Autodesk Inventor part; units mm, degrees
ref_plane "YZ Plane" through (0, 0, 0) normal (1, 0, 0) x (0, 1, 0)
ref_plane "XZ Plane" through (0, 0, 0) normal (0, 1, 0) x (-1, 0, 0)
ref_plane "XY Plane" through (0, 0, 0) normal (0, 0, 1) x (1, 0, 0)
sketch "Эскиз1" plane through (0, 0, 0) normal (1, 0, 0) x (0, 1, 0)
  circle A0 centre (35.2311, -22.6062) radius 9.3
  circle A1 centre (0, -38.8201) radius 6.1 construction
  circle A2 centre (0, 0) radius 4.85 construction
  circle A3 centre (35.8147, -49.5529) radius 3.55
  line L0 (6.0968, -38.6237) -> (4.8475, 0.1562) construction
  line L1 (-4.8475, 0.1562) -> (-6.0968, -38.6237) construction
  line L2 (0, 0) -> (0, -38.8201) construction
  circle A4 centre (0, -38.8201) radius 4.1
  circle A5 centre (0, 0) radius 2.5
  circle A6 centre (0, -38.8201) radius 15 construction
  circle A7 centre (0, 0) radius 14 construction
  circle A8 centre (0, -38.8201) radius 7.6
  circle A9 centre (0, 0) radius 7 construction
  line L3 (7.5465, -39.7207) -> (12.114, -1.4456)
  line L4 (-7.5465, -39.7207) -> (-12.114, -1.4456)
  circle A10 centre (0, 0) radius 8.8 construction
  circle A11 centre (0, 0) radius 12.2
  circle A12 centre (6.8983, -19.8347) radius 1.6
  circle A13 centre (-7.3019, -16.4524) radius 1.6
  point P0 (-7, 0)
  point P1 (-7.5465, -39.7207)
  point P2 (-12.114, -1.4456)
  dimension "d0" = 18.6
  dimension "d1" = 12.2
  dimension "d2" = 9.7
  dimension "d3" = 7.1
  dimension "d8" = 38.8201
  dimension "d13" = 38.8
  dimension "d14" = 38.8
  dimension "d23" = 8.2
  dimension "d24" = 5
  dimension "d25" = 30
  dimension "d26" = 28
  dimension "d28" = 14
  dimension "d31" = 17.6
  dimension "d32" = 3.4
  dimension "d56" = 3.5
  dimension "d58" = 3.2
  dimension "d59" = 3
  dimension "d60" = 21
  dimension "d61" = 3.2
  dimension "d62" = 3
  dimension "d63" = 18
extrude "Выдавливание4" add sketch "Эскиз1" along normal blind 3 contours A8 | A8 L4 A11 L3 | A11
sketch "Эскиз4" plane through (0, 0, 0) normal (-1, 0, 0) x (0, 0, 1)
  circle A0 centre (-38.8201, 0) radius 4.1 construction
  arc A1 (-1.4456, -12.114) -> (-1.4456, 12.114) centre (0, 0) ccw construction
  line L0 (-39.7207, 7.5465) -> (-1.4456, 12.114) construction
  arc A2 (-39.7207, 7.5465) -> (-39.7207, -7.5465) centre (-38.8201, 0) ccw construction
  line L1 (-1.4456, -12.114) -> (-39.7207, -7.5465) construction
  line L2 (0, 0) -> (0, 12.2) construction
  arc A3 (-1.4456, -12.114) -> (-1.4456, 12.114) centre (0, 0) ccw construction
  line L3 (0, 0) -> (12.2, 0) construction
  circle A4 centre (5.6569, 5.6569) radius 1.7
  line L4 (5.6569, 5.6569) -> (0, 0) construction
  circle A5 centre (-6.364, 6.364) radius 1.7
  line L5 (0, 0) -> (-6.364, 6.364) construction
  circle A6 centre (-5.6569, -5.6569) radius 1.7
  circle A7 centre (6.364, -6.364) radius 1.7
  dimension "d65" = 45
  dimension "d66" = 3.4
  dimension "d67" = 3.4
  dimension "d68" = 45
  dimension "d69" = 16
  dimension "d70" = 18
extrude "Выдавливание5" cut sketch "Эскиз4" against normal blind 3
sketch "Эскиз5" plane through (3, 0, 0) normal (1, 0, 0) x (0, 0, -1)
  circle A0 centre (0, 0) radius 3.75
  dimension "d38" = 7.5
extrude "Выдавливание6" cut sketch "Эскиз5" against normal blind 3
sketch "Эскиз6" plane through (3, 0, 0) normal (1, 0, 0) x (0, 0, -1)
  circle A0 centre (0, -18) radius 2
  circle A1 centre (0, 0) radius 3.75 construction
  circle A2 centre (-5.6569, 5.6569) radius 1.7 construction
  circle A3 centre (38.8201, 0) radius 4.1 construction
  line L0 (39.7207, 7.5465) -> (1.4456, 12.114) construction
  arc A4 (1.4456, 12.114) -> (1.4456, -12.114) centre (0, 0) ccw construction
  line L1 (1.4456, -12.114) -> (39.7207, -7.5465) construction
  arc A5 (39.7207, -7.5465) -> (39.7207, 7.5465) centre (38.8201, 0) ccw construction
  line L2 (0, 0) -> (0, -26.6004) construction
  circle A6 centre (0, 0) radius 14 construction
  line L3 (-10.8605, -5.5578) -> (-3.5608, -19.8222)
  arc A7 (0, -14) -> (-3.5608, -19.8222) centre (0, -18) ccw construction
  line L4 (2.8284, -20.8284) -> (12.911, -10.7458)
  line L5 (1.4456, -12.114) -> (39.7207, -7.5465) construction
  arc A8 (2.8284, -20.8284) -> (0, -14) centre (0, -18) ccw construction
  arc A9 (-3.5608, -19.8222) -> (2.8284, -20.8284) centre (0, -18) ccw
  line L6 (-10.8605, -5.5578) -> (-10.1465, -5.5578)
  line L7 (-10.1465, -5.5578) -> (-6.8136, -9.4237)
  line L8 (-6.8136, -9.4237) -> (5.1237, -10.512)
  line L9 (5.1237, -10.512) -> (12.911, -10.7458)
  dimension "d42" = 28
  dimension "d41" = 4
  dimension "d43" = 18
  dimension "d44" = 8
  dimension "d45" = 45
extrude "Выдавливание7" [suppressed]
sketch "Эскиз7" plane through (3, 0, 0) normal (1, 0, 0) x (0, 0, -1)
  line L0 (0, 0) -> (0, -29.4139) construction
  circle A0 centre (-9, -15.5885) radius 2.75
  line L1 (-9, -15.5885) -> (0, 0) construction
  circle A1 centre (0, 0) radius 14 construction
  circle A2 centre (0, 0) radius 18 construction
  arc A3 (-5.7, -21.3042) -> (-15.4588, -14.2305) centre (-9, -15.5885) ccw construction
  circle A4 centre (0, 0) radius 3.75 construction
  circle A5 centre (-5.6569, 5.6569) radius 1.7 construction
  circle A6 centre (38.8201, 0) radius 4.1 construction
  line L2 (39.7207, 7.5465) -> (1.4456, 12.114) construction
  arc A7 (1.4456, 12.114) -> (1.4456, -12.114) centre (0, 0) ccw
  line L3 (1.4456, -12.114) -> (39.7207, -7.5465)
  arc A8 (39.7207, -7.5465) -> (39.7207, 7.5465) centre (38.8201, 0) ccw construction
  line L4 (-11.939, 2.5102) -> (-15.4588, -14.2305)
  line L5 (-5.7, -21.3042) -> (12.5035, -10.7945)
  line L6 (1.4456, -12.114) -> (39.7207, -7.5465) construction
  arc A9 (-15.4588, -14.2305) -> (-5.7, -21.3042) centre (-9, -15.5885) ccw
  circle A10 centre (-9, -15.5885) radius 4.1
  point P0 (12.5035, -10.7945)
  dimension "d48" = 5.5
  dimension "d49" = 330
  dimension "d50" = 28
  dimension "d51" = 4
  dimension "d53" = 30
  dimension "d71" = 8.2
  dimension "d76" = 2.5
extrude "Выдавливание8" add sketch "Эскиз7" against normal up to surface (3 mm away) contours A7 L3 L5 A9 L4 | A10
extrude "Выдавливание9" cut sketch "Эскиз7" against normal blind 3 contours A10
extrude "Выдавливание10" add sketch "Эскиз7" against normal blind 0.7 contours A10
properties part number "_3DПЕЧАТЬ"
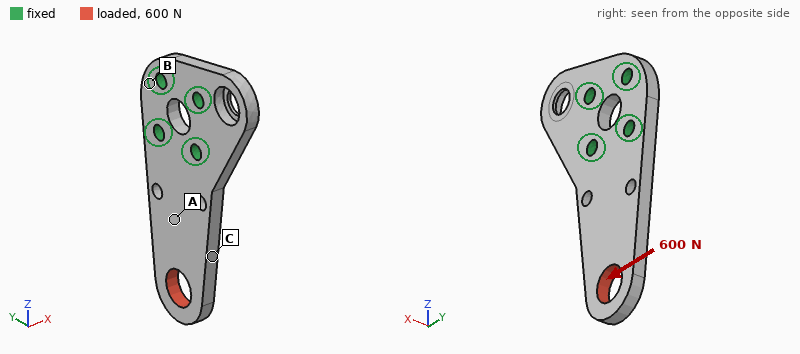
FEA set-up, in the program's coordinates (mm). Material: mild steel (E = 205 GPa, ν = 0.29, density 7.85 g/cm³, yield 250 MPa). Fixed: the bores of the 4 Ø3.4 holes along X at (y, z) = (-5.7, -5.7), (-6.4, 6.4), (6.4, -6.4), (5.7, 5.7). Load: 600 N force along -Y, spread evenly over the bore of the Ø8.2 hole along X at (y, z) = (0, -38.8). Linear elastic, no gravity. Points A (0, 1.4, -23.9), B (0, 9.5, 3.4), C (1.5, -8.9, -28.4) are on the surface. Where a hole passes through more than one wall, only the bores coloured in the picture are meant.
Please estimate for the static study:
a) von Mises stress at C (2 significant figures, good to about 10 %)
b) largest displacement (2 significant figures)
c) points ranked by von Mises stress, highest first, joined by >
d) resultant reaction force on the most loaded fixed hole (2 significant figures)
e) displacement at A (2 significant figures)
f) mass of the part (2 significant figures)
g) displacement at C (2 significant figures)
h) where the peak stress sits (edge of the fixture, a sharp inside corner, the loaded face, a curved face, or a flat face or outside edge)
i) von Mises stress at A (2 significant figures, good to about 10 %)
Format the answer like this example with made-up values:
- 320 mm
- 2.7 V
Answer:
- 47 MPa
- 33 µm
- C > A > B
- 1.2 kN
- 8.1 µm
- 26 g
- 14 µm
- a curved face
- 26 MPa
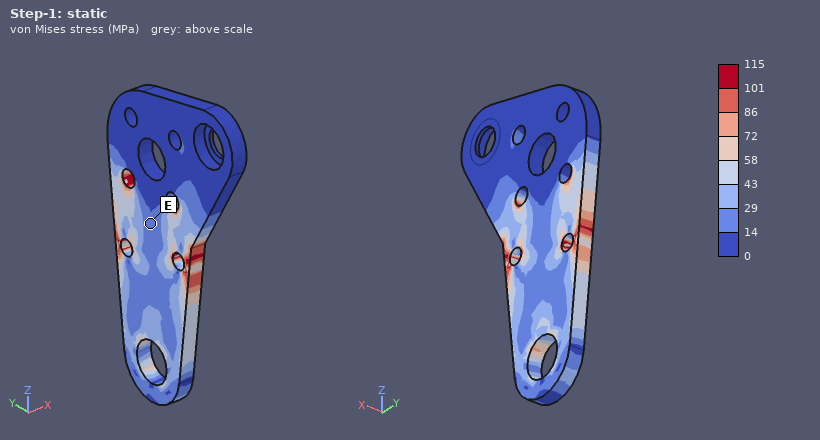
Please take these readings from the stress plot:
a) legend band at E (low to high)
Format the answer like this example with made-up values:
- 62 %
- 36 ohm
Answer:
- 14 to 29 MPa
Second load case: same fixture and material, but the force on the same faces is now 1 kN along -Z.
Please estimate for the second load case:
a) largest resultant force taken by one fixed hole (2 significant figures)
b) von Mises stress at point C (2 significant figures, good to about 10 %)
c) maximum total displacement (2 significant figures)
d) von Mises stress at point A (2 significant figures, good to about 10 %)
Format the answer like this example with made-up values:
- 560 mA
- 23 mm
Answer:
- 470 N
- 22 MPa
- 5.1 µm
- 19 MPa
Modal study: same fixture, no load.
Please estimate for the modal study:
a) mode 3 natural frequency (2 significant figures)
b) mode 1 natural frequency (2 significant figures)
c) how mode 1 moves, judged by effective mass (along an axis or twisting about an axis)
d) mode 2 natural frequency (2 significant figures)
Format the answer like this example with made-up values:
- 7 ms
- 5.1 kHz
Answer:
- 11 kHz
- 2100 Hz
- along X
- 8900 Hz
